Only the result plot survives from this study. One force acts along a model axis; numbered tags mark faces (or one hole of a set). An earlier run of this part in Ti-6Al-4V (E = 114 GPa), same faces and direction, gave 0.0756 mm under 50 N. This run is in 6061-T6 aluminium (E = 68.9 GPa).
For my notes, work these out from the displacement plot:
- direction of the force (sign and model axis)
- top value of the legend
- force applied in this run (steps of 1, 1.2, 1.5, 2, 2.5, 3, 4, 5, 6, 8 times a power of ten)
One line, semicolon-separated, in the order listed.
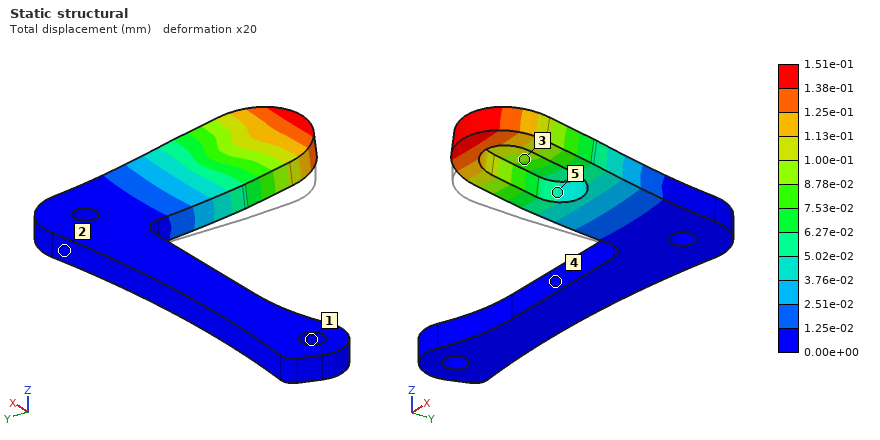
+Z; 1.51e-01 mm; 60 N
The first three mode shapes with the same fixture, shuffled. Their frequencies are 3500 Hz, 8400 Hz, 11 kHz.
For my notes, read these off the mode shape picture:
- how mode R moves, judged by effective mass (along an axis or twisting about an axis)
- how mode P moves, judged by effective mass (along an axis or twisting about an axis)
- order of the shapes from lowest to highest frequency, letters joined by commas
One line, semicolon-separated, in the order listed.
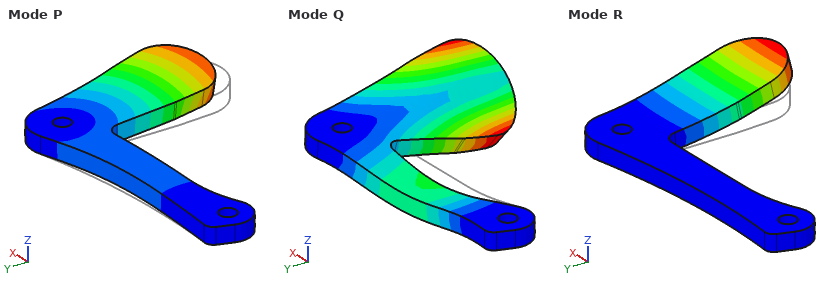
along Z; along X; R, P, Q
